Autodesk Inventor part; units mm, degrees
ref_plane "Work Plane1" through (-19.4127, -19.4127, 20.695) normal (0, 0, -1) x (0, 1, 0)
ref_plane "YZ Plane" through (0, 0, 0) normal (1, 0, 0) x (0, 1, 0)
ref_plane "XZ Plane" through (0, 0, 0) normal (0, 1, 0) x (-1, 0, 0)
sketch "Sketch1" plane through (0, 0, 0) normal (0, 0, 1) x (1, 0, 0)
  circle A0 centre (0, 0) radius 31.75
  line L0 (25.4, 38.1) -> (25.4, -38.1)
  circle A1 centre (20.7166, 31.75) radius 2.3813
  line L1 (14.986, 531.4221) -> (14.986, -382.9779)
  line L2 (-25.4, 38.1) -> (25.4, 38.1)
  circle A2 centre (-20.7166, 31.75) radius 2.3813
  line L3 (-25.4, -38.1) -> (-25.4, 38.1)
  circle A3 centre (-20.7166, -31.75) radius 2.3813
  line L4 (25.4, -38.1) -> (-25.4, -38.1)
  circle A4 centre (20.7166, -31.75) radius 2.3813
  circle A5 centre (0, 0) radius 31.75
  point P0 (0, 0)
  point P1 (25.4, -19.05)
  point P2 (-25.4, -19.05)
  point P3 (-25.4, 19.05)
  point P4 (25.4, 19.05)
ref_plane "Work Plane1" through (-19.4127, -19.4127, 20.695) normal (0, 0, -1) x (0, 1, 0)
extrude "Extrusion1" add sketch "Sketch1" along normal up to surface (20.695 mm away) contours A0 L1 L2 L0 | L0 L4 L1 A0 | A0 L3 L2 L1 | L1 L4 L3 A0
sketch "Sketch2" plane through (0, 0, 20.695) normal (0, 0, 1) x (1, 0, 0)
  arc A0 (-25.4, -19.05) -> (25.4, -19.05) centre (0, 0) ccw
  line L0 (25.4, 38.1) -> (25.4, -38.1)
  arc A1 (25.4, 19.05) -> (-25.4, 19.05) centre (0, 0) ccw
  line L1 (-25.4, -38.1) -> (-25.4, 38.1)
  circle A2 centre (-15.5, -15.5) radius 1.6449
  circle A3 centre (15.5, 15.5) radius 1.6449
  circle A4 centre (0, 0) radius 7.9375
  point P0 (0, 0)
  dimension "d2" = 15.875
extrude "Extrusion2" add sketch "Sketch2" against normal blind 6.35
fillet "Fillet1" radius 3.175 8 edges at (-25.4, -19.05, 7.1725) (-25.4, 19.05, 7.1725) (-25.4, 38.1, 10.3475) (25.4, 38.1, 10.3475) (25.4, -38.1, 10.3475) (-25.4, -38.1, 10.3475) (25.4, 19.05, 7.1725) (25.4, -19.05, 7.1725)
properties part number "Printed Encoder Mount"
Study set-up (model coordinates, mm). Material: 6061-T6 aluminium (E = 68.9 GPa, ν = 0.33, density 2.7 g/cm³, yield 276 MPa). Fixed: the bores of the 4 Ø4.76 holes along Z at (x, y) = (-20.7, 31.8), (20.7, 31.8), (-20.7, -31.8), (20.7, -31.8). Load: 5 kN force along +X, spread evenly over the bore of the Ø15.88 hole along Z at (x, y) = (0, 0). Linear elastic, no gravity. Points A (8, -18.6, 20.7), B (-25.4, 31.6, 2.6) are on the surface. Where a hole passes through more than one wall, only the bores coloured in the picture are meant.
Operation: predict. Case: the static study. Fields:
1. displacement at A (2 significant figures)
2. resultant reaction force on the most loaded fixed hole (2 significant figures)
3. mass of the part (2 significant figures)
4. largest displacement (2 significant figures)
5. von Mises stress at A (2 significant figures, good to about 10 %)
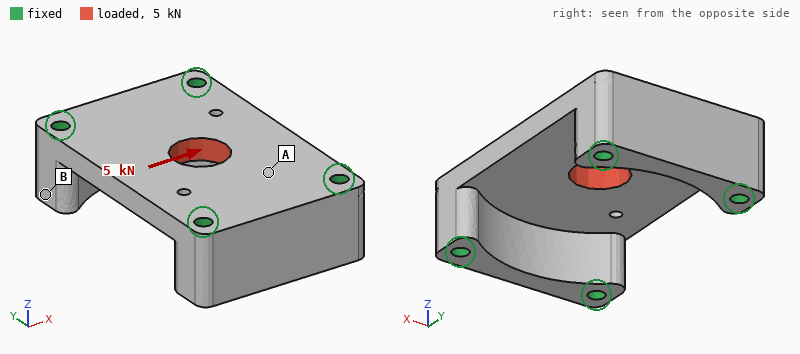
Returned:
4.9 µm
1.6 kN
96 g
12 µm
16 MPa
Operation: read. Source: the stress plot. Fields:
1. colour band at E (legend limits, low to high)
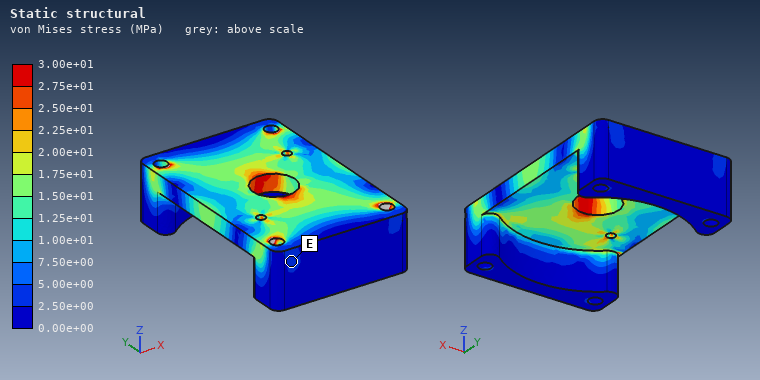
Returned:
2.50e+00 to 5.00e+00 MPa
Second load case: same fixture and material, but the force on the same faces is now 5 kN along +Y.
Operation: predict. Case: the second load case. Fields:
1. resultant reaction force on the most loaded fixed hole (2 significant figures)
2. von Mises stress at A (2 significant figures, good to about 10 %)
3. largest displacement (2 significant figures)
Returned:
1.3 kN
9.6 MPa
6.4 µm
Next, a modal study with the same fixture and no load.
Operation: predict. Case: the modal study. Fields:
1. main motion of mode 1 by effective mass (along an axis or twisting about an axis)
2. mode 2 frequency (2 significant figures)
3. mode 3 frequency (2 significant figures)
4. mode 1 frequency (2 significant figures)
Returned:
along Z
12 kHz
18 kHz
8600 Hz
